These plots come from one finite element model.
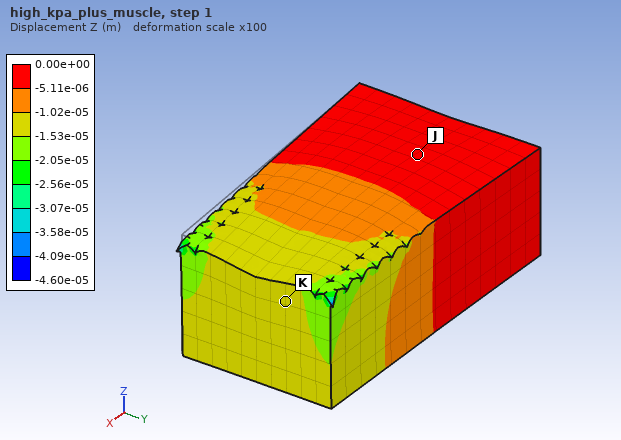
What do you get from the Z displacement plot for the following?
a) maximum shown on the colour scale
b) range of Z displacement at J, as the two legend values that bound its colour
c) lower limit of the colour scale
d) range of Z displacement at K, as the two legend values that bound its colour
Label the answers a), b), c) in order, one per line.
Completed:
a) 0.00e+00 m
b) -5.11e-06 to 0.00e+00 m
c) -4.60e-05 m
d) -1.53e-05 to -1.02e-05 m
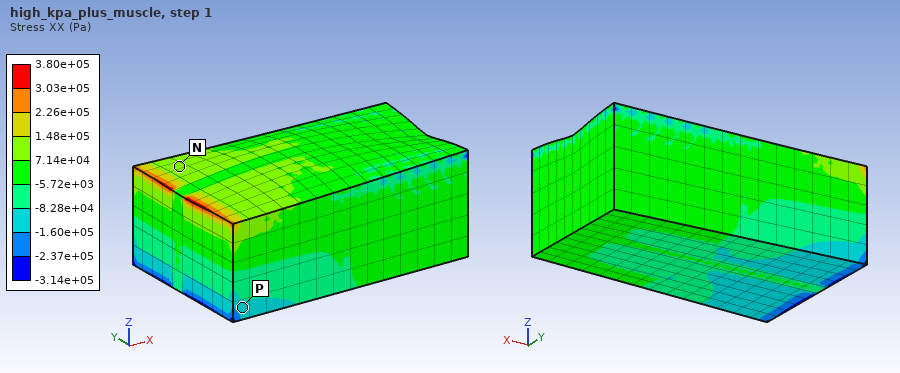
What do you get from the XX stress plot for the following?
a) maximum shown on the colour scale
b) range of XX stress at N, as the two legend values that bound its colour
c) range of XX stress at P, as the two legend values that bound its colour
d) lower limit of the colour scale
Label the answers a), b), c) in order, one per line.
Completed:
a) 3.80e+05 Pa
b) 7.14e+04 to 1.48e+05 Pa
c) -1.60e+05 to -8.28e+04 Pa
d) -3.14e+05 Pa
